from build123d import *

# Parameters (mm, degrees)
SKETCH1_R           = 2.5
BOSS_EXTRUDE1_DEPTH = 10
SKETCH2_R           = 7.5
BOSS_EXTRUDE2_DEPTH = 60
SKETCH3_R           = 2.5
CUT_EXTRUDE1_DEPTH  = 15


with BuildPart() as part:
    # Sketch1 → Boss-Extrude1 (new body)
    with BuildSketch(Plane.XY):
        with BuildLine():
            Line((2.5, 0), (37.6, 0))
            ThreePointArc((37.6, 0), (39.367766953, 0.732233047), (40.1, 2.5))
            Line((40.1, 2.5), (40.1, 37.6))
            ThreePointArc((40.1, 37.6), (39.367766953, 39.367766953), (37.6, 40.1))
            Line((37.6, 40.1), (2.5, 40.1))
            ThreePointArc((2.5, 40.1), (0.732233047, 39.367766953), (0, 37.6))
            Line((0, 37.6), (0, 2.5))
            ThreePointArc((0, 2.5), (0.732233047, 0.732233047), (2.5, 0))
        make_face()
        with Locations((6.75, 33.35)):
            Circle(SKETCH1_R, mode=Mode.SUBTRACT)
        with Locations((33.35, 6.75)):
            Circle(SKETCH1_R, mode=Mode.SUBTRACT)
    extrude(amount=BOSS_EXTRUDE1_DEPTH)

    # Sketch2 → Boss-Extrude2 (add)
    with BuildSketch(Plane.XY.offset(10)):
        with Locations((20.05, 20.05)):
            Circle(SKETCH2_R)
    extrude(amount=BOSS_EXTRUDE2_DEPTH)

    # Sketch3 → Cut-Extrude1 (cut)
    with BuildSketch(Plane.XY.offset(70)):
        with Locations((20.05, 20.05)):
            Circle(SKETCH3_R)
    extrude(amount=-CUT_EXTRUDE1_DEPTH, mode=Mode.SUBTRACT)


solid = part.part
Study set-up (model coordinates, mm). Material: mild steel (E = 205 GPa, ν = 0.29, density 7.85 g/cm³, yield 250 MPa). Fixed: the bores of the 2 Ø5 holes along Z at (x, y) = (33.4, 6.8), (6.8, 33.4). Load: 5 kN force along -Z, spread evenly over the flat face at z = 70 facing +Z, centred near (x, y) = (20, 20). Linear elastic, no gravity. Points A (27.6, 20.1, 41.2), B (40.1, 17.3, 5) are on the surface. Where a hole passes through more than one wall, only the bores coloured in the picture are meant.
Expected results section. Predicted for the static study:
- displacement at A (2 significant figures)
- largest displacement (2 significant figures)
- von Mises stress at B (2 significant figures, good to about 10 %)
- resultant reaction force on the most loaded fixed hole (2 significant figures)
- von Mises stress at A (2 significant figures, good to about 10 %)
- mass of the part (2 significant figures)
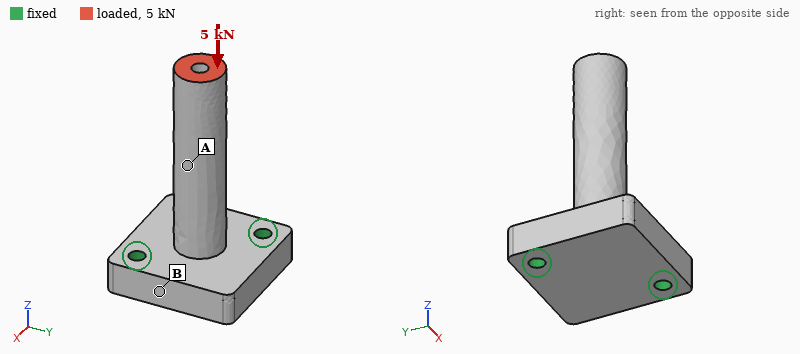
8.9 µm
13 µm
14 MPa
2.5 kN
28 MPa
200 g
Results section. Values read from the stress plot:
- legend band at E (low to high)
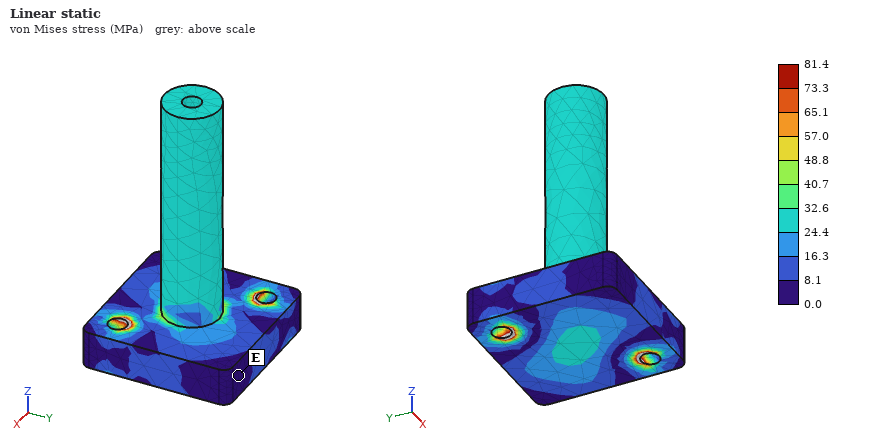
0.0 to 8.1 MPa
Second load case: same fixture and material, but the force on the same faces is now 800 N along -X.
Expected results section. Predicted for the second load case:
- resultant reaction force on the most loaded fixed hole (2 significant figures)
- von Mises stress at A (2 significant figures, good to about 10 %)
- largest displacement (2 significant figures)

1.3 kN
69 MPa
0.16 mm
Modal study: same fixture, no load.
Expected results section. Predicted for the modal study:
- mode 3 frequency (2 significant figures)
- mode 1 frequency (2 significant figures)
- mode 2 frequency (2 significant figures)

11 kHz
2300 Hz
2600 Hz
